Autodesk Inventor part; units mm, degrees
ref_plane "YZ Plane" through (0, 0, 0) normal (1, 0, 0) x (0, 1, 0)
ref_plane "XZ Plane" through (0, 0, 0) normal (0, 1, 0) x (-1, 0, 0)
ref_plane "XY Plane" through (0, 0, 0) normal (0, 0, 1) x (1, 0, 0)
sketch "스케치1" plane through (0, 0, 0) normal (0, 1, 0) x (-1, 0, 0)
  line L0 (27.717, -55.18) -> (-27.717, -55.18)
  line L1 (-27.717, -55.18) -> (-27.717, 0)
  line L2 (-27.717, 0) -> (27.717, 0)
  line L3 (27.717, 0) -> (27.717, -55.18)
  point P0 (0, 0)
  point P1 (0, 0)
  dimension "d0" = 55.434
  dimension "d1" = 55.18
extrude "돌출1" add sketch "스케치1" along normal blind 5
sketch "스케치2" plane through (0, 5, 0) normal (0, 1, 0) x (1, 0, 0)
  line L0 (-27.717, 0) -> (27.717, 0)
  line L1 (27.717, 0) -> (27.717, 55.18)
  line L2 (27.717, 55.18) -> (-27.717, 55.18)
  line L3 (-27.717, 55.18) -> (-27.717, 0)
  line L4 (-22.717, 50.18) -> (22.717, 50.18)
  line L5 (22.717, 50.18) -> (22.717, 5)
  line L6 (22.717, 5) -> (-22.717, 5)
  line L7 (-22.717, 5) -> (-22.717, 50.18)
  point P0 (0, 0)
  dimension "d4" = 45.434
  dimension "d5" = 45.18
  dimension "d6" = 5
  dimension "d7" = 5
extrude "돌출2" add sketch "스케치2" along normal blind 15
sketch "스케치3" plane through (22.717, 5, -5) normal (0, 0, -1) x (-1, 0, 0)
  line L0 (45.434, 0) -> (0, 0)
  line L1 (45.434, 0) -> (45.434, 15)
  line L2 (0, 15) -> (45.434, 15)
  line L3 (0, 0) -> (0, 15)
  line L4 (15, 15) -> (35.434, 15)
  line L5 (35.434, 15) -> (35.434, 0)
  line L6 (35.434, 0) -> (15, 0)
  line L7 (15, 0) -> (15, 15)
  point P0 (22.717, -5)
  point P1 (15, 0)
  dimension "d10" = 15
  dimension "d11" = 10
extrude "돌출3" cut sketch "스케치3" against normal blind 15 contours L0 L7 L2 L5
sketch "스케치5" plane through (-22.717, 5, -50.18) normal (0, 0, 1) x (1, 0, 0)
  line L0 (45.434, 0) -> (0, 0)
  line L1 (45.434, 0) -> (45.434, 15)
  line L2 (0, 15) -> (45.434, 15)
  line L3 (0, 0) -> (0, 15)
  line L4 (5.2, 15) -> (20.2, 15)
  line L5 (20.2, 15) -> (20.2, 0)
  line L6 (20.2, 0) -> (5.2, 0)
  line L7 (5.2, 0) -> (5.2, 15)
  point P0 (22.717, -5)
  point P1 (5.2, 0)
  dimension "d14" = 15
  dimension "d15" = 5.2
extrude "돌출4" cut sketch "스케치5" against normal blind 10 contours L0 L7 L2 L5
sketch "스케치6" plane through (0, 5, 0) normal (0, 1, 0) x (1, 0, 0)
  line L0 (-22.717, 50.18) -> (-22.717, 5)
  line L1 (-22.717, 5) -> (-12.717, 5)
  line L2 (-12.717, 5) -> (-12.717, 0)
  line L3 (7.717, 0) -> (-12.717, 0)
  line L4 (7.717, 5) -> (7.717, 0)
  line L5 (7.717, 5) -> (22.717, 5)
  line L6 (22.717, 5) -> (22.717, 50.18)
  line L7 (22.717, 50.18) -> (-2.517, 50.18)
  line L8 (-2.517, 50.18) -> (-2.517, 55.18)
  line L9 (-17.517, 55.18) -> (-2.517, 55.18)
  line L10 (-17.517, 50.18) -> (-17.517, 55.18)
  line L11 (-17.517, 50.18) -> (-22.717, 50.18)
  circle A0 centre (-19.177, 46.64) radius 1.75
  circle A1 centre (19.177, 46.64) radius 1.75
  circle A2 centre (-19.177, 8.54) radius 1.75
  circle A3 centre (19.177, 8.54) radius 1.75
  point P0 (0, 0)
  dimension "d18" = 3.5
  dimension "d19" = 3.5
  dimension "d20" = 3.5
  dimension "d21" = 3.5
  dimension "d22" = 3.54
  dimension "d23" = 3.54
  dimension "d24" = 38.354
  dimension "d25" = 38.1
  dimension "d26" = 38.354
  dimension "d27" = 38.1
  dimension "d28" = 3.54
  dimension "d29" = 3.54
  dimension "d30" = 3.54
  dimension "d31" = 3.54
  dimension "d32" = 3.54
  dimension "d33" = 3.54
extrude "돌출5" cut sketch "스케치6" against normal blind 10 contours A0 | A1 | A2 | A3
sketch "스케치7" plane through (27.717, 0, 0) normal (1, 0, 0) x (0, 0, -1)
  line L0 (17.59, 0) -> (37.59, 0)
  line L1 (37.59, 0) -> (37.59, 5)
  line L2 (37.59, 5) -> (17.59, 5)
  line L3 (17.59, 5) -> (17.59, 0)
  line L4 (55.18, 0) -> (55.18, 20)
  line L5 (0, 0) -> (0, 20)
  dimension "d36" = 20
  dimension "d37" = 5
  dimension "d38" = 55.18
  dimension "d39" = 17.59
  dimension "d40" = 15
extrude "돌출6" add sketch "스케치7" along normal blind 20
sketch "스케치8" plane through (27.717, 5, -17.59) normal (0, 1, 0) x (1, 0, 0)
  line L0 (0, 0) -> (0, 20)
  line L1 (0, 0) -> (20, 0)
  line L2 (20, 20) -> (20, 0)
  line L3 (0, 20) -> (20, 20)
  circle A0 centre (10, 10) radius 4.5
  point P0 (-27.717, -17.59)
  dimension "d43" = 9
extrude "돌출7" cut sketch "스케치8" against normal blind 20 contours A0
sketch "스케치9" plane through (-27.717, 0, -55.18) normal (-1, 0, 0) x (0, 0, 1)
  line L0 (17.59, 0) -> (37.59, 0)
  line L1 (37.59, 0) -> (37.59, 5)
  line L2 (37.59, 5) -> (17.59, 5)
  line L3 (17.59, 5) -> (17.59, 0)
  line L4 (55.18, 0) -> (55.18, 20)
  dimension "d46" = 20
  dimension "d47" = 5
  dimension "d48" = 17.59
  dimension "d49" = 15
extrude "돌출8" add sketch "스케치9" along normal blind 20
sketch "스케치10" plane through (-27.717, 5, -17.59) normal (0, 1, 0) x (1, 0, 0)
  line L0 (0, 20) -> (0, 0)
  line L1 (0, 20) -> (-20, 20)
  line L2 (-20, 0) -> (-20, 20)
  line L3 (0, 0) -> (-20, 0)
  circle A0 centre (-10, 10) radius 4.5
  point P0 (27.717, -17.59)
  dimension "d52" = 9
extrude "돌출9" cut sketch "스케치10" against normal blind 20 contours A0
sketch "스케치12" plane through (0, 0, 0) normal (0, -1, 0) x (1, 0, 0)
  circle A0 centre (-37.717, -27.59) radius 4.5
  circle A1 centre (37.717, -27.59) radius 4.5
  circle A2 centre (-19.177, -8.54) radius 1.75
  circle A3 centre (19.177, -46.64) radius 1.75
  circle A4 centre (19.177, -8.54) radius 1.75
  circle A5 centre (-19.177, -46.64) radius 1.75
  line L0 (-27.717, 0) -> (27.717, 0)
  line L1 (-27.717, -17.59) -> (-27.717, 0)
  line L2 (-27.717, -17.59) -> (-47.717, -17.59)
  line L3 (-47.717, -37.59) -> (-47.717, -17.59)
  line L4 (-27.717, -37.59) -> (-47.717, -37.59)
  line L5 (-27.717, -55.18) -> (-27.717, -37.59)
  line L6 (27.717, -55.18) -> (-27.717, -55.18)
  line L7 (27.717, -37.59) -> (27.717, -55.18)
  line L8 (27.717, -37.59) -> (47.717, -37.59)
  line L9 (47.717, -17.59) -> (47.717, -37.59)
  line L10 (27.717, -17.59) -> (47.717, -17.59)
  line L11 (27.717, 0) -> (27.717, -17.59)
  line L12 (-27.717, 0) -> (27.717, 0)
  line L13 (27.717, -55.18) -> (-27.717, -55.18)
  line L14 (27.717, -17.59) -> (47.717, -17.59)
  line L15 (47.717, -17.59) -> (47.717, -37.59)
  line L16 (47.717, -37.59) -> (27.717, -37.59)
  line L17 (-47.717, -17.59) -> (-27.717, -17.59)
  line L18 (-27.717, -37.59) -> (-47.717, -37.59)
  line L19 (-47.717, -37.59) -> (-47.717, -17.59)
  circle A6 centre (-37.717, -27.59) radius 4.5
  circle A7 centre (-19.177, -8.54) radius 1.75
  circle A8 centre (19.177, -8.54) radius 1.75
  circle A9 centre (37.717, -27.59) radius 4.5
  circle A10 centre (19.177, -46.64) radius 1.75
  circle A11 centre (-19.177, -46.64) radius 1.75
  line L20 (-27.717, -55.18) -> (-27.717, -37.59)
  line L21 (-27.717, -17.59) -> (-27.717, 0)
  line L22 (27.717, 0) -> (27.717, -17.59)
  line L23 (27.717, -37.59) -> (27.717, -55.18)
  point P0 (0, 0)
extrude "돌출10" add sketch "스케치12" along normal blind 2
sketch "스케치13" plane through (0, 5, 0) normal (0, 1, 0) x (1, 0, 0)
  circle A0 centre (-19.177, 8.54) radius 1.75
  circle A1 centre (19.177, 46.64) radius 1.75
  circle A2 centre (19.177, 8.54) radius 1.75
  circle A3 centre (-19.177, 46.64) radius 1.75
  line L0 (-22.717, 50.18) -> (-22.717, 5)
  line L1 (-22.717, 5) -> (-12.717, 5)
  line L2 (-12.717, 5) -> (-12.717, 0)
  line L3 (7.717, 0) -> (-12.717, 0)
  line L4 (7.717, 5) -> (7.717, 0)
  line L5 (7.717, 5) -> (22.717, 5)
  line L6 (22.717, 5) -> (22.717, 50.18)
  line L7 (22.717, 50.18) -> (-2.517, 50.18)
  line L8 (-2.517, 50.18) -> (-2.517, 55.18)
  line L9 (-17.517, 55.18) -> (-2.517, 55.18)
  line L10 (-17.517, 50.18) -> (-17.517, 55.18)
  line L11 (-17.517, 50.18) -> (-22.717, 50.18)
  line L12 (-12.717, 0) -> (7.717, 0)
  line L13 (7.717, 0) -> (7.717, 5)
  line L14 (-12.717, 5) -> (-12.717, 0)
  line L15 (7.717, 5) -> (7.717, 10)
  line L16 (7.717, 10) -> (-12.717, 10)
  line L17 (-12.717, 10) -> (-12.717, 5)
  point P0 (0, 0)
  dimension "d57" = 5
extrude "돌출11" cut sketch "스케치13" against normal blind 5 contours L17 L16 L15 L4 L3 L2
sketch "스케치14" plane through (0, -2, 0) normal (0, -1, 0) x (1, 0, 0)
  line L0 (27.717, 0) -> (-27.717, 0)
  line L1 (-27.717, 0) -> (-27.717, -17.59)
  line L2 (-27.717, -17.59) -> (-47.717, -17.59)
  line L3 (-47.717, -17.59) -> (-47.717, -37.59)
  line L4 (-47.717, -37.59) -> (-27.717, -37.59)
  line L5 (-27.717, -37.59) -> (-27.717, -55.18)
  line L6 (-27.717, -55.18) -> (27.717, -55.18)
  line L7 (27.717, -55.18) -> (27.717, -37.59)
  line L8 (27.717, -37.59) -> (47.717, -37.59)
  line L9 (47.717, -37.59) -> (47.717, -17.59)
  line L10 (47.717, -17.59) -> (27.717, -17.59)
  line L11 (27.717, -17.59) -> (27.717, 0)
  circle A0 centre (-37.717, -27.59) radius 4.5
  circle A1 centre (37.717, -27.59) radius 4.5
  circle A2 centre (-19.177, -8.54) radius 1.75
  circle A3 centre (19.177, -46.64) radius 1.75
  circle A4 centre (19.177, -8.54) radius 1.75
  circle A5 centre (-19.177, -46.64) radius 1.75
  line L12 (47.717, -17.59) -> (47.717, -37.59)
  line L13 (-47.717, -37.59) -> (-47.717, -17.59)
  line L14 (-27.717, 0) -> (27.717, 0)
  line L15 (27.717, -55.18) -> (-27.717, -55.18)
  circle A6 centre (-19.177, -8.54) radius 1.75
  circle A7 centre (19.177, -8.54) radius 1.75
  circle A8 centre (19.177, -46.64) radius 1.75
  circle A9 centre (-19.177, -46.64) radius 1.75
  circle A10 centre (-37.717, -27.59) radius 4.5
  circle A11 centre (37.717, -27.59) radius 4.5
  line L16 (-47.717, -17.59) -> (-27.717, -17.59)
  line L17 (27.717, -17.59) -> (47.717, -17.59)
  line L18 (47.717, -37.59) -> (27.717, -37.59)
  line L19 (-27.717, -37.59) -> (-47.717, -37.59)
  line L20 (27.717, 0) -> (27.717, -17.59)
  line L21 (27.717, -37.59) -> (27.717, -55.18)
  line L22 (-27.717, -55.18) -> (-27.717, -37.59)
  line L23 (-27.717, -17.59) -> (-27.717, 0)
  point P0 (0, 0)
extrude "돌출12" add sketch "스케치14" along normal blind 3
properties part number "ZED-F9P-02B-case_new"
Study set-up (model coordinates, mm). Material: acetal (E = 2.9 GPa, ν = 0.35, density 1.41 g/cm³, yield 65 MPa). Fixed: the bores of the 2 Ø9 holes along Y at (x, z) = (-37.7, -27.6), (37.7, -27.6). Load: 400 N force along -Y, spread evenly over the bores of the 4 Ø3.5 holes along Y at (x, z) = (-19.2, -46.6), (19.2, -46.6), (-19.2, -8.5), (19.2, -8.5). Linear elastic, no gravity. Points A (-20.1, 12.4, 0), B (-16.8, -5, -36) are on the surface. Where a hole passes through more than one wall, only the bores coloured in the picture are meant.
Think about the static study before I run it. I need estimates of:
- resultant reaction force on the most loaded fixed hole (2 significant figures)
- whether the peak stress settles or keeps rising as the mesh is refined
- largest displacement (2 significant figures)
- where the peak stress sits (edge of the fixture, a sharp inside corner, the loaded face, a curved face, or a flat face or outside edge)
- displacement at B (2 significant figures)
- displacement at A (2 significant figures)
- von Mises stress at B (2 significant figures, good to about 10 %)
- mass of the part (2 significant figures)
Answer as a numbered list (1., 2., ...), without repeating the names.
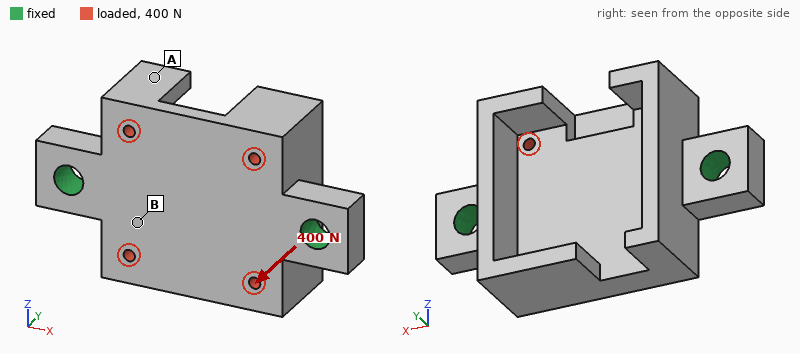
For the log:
1. 200 N
2. keeps rising
3. 91 µm
4. edge of the fixture
5. 45 µm
6. 63 µm
7. 1.7 MPa
8. 68 g
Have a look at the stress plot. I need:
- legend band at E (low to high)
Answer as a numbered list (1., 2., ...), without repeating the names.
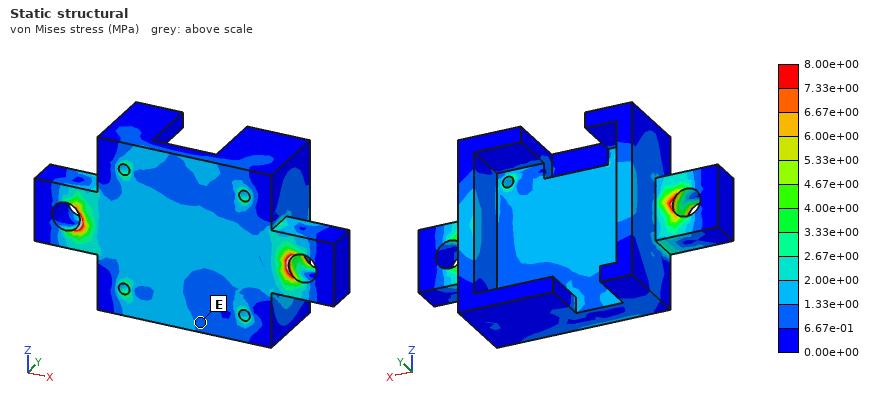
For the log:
1. 6.67e-01 to 1.33e+00 MPa
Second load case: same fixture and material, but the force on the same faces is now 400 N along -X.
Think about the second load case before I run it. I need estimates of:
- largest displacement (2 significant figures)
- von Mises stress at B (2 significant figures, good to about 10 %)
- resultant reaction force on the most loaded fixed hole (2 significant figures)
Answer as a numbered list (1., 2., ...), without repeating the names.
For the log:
1. 13 µm
2. 0.70 MPa
3. 200 N
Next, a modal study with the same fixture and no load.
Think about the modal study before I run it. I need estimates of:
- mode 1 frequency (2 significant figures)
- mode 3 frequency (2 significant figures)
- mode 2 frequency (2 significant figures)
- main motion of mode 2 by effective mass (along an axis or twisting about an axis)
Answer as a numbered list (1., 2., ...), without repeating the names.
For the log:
1. 1100 Hz
2. 2200 Hz
3. 1700 Hz
4. along Y
